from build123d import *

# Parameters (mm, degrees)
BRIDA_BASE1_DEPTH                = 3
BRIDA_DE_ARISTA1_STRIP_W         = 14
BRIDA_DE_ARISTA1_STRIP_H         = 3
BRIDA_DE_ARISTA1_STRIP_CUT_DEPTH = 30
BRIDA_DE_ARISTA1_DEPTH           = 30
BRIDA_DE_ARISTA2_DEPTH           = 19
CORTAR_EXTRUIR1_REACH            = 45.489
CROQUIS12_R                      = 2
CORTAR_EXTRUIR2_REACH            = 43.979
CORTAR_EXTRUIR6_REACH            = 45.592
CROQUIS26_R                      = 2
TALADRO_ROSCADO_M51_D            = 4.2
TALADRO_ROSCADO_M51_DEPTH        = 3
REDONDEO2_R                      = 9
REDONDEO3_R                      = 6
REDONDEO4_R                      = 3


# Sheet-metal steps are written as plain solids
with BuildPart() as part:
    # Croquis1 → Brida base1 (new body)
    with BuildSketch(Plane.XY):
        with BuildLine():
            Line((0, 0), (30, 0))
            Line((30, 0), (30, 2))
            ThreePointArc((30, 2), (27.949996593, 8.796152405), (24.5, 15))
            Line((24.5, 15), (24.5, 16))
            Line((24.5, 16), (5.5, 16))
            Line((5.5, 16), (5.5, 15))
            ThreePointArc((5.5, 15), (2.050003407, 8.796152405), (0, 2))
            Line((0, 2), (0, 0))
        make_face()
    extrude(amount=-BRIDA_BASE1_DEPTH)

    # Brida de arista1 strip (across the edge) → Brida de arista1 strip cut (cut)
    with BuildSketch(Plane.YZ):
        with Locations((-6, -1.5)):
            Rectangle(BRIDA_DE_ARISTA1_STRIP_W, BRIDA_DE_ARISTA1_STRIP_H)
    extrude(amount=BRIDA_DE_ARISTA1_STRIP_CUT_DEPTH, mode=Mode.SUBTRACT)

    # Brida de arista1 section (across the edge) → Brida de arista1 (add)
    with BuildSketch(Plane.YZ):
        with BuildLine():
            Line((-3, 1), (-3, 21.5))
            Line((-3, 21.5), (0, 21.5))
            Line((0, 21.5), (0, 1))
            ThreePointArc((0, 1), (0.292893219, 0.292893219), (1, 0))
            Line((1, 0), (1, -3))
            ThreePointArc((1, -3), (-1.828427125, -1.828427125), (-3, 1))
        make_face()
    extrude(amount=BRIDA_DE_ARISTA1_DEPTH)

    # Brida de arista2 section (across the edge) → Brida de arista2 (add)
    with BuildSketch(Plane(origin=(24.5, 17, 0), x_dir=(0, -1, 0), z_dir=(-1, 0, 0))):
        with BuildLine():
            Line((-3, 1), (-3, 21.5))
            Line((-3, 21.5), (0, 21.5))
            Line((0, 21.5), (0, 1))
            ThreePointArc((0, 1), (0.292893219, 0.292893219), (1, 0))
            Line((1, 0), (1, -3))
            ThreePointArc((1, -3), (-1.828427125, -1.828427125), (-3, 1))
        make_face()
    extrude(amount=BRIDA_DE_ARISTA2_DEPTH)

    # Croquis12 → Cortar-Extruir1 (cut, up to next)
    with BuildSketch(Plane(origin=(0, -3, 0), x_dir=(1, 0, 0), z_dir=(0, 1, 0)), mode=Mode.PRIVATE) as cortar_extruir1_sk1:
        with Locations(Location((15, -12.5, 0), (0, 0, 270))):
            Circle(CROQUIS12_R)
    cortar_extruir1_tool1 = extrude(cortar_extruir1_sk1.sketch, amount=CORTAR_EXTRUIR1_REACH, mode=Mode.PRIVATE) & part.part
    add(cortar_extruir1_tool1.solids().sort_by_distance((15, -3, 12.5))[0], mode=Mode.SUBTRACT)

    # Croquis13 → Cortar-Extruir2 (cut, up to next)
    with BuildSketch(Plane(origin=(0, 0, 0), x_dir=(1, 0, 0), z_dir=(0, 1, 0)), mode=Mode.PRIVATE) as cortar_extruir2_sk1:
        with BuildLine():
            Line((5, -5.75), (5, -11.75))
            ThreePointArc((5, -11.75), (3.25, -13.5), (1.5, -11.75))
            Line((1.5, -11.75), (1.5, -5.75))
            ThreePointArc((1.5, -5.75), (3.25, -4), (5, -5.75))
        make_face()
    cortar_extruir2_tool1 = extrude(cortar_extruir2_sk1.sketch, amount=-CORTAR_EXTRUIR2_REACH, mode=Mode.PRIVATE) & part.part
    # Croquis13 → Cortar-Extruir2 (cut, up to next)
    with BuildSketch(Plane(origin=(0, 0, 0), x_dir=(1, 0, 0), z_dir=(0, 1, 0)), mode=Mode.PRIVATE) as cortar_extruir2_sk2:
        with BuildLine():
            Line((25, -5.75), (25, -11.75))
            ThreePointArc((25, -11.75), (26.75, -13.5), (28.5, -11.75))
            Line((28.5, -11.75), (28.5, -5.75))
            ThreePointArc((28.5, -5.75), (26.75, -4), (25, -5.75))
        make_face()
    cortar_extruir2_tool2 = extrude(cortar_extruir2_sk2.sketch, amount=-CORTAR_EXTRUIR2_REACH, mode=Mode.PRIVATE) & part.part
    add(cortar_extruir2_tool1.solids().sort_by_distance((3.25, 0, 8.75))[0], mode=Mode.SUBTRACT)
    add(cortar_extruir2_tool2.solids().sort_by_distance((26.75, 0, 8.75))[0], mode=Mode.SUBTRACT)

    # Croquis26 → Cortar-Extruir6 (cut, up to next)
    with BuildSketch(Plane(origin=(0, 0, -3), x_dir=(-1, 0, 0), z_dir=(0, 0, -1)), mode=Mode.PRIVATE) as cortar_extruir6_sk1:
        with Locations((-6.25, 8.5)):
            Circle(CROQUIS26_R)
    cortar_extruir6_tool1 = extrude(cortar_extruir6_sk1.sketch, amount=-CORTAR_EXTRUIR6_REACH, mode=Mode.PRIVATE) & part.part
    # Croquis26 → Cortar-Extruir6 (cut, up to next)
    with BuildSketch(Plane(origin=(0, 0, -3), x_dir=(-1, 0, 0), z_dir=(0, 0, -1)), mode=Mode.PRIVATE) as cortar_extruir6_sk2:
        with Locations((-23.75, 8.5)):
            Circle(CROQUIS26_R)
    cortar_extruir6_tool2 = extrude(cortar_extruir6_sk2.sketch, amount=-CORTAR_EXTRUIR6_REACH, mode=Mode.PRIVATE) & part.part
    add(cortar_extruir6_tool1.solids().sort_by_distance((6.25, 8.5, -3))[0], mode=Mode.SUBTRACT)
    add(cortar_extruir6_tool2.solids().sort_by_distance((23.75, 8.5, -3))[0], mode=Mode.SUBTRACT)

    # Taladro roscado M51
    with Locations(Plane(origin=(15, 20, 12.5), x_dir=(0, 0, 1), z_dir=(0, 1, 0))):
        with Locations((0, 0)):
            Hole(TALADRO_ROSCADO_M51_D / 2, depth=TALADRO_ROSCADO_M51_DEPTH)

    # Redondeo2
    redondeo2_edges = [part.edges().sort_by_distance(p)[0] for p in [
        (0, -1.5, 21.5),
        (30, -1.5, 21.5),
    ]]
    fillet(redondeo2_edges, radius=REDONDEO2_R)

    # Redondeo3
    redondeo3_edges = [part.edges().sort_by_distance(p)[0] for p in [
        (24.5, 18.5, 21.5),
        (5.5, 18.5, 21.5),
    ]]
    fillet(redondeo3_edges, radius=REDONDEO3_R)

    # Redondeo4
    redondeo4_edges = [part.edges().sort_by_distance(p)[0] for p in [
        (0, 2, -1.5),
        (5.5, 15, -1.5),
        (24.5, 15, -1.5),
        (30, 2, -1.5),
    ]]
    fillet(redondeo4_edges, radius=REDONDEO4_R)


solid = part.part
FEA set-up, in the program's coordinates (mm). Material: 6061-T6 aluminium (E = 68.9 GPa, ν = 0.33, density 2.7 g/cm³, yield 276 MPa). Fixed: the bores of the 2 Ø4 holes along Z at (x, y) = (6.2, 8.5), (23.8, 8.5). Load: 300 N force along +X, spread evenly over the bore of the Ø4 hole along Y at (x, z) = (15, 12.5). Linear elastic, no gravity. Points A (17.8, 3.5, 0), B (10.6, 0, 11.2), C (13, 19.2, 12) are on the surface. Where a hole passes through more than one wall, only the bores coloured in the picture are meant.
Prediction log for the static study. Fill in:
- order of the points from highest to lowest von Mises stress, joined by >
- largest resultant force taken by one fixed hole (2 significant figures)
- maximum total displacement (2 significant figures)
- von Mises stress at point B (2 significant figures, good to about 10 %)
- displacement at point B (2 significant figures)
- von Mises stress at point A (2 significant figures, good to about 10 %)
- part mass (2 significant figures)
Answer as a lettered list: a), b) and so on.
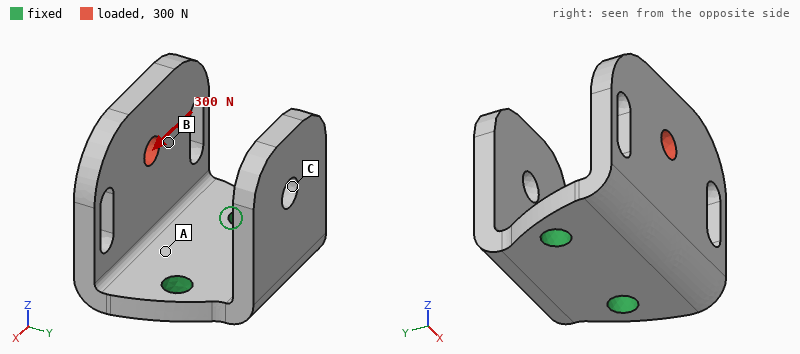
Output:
a) A > B > C
b) 290 N
c) 48 µm
d) 14 MPa
e) 27 µm
f) 33 MPa
g) 11 g
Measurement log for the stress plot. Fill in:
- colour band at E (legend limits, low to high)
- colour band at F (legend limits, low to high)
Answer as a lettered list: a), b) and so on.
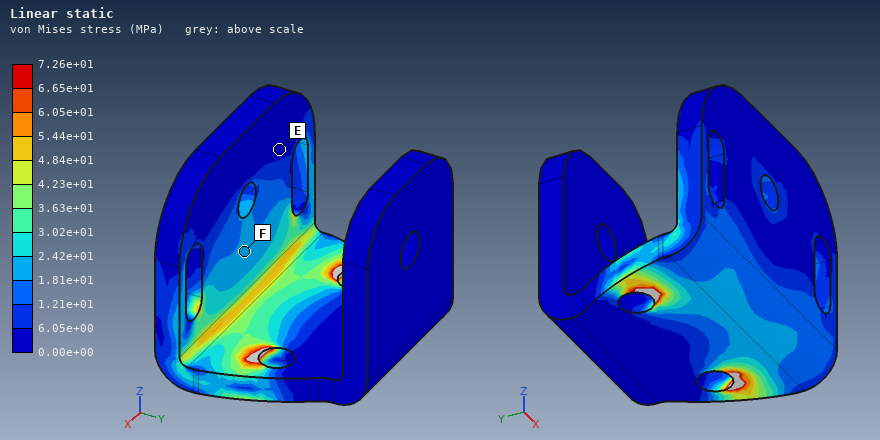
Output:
a) 0.00e+00 to 6.05e+00 MPa
b) 1.81e+01 to 2.42e+01 MPa
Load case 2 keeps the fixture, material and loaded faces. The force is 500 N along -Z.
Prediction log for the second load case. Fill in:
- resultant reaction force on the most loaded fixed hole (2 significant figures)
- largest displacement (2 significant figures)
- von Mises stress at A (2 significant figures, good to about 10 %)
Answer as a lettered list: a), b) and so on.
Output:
a) 250 N
b) 0.12 mm
c) 44 MPa
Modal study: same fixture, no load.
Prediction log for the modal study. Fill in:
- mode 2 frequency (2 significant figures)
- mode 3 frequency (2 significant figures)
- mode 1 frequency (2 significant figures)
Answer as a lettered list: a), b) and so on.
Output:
a) 3200 Hz
b) 6700 Hz
c) 3100 Hz
